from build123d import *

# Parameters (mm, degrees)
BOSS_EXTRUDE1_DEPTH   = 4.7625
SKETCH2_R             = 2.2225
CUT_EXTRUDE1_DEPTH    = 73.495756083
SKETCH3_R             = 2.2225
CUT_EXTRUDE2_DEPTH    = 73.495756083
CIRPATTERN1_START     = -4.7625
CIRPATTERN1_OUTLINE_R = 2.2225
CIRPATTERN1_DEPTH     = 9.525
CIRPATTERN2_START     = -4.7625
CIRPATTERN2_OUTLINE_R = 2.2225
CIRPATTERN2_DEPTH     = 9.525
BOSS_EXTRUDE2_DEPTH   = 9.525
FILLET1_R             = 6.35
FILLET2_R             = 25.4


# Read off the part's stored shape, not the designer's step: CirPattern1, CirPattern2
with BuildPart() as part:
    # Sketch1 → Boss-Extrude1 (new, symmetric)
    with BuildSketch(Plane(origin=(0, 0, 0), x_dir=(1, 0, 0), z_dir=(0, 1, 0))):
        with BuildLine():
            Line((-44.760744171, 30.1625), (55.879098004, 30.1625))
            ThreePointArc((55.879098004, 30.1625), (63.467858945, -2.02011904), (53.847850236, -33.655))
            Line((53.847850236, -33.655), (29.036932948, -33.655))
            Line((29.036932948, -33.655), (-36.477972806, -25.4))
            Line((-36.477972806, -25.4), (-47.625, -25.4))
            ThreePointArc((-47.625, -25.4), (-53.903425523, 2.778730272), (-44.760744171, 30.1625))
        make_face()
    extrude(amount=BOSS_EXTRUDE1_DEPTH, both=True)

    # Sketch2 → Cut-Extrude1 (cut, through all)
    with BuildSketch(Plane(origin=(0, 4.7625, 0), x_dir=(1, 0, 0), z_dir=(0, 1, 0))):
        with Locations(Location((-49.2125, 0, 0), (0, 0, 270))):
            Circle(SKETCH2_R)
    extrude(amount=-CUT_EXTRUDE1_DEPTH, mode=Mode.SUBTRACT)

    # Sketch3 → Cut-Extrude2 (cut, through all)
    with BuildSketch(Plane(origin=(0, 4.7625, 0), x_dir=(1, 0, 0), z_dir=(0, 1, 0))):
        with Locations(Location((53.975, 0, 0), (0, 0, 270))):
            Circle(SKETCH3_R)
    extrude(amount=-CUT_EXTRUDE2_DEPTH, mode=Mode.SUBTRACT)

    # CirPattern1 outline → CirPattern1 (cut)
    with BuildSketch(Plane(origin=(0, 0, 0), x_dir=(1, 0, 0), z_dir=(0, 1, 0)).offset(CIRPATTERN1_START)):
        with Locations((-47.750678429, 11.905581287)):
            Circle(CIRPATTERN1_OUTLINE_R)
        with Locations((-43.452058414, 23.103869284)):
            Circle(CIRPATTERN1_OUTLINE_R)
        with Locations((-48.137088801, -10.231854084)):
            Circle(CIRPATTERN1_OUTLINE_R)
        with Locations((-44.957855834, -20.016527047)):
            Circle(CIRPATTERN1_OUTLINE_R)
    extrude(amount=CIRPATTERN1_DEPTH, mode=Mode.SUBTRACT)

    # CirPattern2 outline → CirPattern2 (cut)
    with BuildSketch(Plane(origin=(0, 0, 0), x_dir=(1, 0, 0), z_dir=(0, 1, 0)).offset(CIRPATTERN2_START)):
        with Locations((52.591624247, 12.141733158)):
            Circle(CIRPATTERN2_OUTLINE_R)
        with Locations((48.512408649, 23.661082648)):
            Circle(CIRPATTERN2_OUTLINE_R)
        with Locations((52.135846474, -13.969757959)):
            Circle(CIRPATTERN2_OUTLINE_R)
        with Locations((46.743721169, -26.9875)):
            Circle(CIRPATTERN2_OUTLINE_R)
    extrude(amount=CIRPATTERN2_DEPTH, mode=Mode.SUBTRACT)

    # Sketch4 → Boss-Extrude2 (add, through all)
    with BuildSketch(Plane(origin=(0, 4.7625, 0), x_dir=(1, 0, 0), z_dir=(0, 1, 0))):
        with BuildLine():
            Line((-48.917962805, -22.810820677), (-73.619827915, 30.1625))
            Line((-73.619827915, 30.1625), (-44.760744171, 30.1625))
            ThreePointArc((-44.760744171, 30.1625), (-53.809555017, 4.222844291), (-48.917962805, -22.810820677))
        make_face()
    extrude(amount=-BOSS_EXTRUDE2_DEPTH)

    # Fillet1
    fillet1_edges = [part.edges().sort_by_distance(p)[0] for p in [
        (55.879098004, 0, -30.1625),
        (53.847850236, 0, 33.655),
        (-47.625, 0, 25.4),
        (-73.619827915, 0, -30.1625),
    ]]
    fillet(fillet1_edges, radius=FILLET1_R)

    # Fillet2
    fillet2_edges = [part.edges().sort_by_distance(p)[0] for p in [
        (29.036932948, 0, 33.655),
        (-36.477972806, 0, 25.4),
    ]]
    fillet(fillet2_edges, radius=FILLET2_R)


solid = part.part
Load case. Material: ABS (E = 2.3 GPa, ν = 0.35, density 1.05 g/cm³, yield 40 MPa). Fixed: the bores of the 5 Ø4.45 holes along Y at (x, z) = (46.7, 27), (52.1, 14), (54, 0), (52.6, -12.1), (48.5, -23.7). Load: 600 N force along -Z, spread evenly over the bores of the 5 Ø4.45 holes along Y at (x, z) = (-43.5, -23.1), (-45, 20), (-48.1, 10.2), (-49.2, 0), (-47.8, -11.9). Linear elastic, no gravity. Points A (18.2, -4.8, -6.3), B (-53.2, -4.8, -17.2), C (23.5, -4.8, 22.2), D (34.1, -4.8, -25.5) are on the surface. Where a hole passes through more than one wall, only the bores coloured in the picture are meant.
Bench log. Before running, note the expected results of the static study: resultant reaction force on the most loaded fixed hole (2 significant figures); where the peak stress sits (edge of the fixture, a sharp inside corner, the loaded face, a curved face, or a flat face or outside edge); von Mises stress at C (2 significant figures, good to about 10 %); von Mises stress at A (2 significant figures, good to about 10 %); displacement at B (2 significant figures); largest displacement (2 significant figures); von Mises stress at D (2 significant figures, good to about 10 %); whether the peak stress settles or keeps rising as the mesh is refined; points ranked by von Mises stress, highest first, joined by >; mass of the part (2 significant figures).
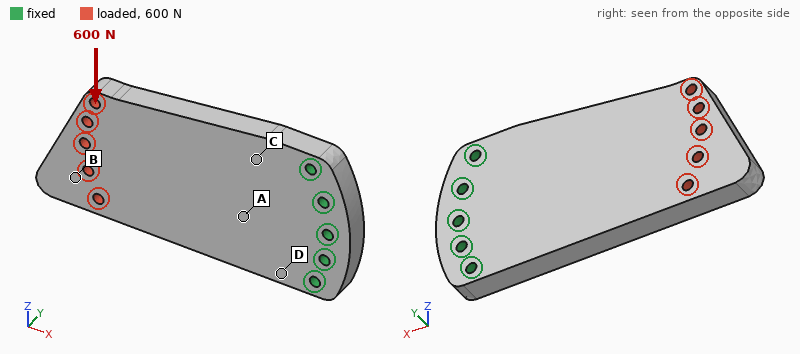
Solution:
1.0 kN
edge of the fixture
4.9 MPa
2.7 MPa
0.57 mm
0.69 mm
6.7 MPa
keeps rising
D > C > A > B
71 g
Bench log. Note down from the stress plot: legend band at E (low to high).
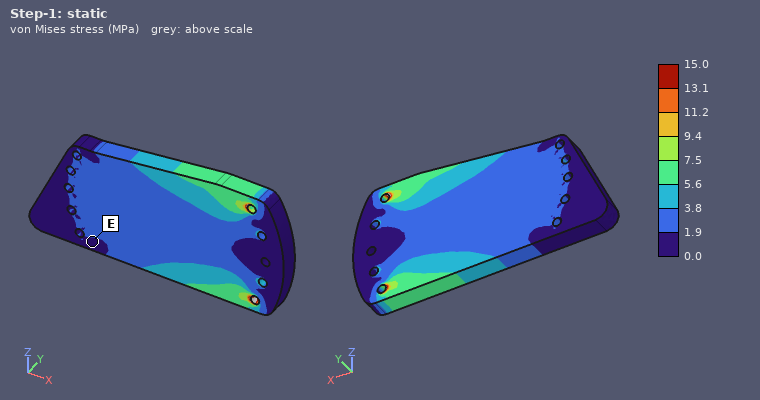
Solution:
0.0 to 1.9 MPa
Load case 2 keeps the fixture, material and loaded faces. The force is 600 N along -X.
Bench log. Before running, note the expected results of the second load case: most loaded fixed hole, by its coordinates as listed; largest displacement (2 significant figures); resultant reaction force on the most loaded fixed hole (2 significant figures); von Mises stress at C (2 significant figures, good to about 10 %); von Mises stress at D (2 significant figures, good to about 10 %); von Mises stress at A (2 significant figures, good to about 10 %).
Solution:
(48.5, -23.7)
50 µm
180 N
0.88 MPa
1.2 MPa
1.1 MPa
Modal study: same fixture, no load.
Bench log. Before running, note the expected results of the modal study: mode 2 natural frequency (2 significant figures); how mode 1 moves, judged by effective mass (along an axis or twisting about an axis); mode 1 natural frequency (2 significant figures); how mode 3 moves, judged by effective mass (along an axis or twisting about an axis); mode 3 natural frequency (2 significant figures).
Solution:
800 Hz
along Y
200 Hz
along Z
1100 Hz
